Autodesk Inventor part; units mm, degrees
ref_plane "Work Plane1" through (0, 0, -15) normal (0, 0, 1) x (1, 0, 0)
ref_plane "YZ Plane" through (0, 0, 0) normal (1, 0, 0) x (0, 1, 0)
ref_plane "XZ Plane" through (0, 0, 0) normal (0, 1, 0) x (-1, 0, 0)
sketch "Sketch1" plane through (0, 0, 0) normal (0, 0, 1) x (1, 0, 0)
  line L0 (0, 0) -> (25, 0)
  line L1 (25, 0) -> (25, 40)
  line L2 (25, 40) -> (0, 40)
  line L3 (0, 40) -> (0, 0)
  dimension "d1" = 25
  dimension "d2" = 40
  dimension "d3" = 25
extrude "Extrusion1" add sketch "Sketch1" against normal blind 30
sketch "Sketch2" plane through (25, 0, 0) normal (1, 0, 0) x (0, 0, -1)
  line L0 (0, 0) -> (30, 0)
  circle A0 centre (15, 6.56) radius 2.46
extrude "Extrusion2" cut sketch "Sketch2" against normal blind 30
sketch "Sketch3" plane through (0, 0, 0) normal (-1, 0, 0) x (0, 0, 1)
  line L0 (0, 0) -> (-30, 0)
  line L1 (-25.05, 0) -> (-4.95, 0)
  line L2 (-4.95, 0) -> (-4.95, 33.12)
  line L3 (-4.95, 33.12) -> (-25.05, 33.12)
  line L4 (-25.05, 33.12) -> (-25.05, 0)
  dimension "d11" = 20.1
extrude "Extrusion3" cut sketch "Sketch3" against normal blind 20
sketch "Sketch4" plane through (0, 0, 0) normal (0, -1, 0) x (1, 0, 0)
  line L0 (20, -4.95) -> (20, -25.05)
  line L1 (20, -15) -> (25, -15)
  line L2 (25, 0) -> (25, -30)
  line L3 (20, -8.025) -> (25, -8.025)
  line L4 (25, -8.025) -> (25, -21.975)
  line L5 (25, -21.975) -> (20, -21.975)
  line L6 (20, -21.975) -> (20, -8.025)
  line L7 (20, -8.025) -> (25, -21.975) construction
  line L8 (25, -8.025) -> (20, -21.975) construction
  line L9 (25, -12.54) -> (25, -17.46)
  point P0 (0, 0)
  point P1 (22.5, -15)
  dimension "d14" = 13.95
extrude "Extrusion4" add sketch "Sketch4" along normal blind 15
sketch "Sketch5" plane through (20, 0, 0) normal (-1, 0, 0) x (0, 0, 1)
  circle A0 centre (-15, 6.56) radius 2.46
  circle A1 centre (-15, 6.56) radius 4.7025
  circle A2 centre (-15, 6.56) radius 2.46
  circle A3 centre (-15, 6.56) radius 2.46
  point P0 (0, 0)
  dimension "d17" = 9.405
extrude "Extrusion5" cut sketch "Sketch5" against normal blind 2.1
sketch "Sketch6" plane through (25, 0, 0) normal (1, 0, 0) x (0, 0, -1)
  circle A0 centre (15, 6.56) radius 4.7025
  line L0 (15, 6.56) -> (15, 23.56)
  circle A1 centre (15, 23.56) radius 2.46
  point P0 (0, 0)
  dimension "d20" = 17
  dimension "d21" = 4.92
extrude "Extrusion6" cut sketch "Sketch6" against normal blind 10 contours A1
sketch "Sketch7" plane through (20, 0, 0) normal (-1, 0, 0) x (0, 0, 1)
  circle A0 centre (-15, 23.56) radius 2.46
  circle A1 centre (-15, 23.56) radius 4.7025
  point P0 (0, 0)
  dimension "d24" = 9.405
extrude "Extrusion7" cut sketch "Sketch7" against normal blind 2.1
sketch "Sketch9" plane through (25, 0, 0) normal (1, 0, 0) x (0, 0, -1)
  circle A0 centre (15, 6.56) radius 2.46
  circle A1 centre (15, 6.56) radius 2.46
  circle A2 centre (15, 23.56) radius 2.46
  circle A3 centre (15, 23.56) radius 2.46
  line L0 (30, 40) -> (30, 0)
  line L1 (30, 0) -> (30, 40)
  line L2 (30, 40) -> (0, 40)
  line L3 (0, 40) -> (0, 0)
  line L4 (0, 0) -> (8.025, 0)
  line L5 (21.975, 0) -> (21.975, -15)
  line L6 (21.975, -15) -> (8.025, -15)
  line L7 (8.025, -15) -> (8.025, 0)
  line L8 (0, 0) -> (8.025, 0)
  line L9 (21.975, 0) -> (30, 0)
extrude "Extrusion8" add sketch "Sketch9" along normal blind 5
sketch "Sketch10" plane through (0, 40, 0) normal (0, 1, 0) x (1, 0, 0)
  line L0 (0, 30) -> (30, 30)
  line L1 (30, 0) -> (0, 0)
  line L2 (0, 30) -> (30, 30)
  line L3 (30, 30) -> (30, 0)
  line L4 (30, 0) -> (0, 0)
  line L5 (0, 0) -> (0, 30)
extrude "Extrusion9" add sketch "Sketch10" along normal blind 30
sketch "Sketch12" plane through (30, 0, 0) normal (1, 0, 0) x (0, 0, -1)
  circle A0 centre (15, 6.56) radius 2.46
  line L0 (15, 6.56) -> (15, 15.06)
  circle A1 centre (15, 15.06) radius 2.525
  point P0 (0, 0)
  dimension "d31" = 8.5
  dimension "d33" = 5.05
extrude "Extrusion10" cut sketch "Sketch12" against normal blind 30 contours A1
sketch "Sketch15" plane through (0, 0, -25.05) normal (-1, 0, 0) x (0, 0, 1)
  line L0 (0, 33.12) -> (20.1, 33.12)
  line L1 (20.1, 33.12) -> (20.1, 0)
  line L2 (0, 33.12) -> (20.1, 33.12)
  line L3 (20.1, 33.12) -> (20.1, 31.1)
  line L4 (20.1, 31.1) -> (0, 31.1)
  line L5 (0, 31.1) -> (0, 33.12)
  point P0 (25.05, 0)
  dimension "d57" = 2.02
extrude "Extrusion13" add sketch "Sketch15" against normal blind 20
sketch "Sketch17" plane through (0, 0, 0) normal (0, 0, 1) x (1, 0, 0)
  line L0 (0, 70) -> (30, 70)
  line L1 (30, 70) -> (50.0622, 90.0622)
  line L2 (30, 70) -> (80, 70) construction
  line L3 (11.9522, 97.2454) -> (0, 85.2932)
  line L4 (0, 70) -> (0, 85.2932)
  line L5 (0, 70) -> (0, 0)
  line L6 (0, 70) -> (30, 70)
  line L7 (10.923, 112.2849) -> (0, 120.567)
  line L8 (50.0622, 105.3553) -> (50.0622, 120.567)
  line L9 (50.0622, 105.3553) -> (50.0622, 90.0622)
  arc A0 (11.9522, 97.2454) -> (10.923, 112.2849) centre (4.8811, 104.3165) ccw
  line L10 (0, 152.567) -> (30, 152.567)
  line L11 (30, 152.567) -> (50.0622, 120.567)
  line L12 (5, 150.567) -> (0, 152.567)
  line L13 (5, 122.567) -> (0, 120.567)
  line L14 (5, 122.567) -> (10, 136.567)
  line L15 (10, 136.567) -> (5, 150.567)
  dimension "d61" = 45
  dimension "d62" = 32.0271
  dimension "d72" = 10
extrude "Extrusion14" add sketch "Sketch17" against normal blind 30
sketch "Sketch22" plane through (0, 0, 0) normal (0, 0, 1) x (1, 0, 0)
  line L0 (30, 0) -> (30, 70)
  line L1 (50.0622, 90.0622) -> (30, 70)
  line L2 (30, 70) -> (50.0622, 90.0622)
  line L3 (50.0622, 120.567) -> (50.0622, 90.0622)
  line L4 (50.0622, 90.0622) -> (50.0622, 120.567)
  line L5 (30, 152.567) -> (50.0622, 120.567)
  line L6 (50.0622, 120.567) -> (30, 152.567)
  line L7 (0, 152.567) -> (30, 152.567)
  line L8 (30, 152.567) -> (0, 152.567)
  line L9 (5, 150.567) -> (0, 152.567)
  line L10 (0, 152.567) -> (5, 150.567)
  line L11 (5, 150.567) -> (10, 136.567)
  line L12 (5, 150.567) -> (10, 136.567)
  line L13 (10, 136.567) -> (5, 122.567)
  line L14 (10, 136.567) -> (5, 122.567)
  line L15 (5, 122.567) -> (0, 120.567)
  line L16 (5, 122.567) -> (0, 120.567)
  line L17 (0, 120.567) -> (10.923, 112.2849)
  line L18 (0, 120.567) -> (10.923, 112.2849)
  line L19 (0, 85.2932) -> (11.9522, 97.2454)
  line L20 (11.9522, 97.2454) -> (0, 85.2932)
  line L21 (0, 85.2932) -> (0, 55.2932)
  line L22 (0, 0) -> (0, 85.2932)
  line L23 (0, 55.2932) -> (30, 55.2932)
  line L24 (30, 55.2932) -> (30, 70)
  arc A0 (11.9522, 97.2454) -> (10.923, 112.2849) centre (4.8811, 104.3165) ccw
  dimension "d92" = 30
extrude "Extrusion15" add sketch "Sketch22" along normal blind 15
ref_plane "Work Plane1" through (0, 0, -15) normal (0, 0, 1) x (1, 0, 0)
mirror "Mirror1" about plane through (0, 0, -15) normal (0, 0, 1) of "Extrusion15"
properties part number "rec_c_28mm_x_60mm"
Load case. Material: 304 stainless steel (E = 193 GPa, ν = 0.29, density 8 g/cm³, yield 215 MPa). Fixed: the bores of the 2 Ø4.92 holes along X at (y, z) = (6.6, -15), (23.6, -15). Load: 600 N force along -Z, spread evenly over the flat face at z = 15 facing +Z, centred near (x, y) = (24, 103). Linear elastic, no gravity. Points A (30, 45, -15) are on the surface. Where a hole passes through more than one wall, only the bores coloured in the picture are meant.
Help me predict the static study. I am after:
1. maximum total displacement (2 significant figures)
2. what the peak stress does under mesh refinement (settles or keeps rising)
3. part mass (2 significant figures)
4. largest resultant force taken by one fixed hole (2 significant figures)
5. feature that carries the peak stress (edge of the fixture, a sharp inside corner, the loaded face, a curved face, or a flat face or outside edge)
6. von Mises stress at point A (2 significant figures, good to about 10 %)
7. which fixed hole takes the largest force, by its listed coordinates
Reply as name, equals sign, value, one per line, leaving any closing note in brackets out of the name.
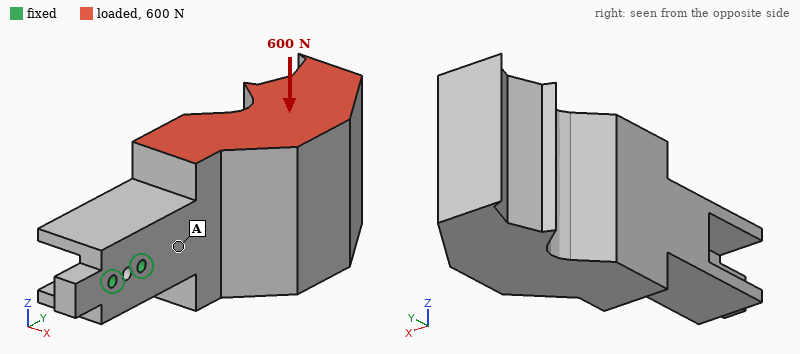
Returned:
maximum total displacement = 46 µm
what the peak stress does under mesh refinement = keeps rising
part mass = 2.0 kg
largest resultant force taken by one fixed hole = 2.7 kN
feature that carries the peak stress = edge of the fixture
von Mises stress at point A = 5.9 MPa
which fixed hole takes the largest force, by its listed coordinates = (23.6, -15)
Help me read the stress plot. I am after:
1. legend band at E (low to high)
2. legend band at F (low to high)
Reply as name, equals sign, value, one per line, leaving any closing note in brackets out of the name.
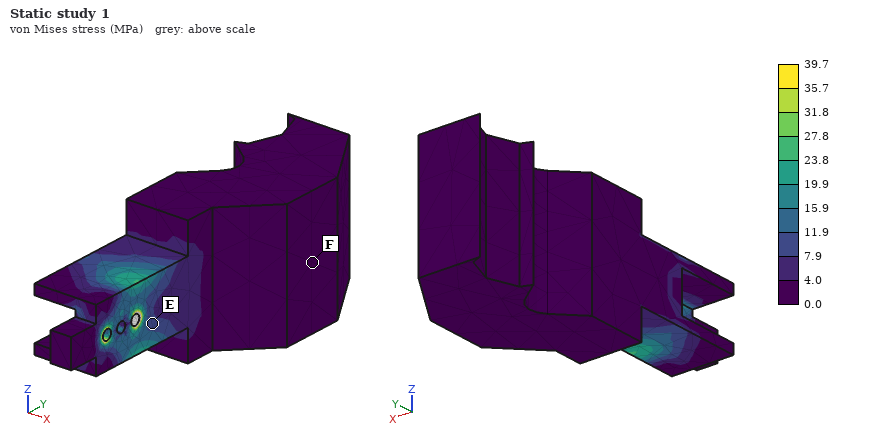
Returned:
legend band at E = 7.9 to 11.9 MPa
legend band at F = 0.0 to 4.0 MPa
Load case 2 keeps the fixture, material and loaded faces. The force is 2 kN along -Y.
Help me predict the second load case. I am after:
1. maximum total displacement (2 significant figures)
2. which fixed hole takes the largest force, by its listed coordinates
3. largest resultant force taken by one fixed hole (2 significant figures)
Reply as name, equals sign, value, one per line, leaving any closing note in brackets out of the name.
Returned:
maximum total displacement = 64 µm
which fixed hole takes the largest force, by its listed coordinates = (23.6, -15)
largest resultant force taken by one fixed hole = 3.0 kN
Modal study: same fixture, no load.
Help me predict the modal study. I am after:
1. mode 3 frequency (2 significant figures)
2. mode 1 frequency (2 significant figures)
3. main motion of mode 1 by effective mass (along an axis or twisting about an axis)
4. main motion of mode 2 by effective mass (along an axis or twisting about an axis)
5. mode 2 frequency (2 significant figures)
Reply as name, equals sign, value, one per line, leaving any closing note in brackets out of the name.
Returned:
mode 3 frequency = 1300 Hz
mode 1 frequency = 460 Hz
main motion of mode 1 by effective mass = along X
main motion of mode 2 by effective mass = along Z
mode 2 frequency = 530 Hz
